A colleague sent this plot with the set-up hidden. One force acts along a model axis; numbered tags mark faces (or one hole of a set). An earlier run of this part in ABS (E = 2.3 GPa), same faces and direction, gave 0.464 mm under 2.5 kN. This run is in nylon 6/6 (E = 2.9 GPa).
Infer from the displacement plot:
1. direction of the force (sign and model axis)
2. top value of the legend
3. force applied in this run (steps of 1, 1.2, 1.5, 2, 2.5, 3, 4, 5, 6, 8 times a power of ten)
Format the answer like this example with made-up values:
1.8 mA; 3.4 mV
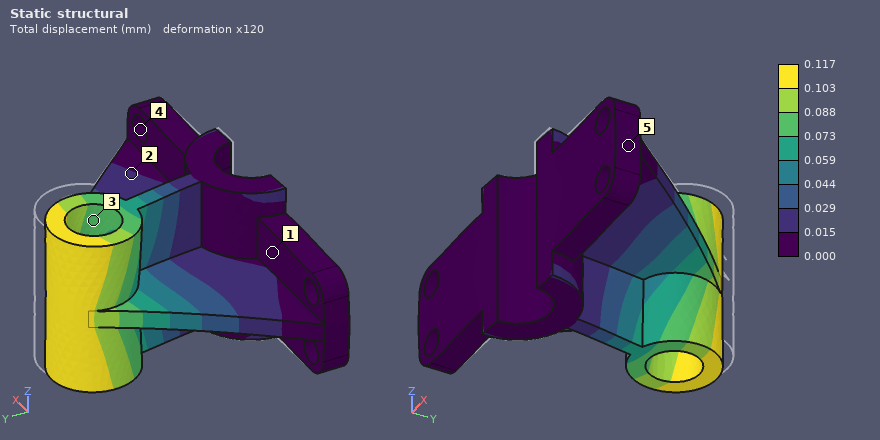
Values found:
-X; 0.117 mm; 800 N
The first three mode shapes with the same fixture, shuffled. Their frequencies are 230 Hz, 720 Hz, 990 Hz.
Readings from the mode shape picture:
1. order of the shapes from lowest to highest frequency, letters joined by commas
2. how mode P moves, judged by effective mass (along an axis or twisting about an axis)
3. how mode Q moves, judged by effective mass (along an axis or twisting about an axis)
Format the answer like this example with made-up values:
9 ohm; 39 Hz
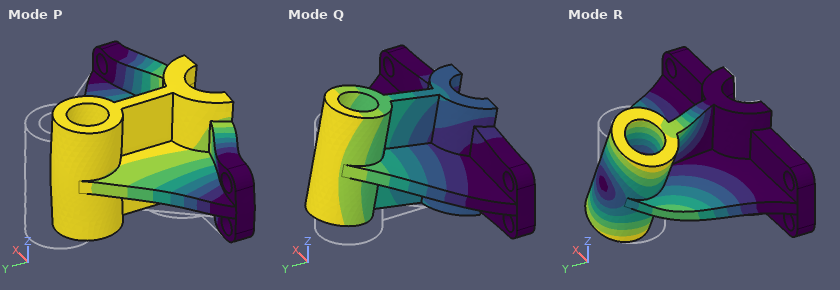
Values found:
Q, R, P; along Y; along Z
